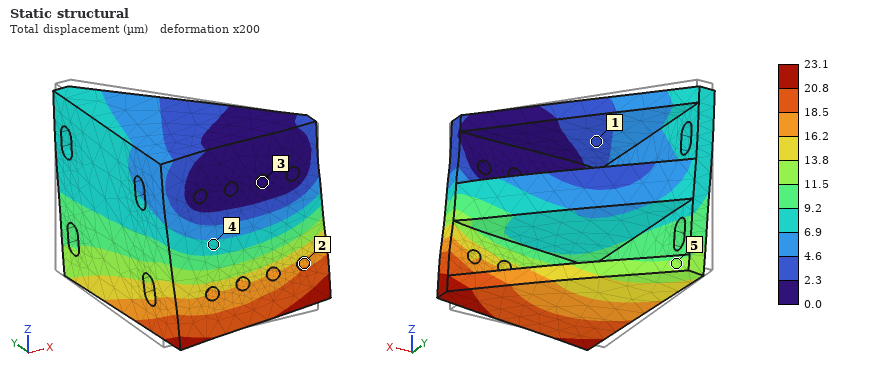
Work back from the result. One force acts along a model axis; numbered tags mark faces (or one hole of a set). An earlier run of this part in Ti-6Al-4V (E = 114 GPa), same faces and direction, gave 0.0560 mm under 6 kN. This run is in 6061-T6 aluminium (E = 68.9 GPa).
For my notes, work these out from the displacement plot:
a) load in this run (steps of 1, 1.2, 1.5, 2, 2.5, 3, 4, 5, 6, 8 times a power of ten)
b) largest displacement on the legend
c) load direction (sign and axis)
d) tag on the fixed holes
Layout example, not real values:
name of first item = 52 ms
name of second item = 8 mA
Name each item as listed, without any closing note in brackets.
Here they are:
load in this run = 1.5 kN
largest displacement on the legend = 23.1 µm
load direction = +X
tag on the fixed holes = 3
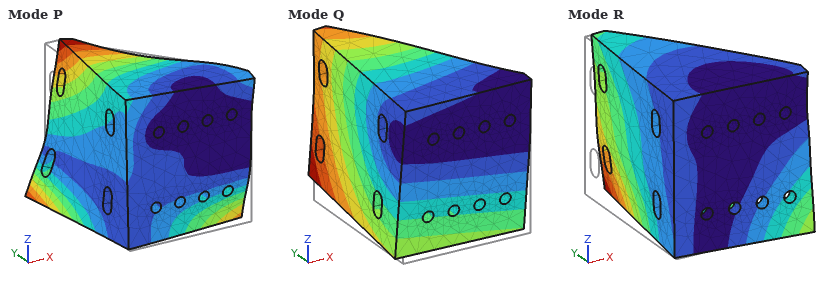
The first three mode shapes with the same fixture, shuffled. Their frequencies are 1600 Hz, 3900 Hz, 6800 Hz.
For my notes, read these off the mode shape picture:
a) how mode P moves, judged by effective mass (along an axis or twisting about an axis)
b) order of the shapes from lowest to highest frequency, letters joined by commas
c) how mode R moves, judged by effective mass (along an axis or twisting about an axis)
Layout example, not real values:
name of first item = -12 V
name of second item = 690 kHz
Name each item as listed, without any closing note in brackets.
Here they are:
how mode P moves, judged by effective mass = along Y
order of the shapes from lowest to highest frequency, letters joined by commas = Q, R, P
how mode R moves, judged by effective mass = along X
